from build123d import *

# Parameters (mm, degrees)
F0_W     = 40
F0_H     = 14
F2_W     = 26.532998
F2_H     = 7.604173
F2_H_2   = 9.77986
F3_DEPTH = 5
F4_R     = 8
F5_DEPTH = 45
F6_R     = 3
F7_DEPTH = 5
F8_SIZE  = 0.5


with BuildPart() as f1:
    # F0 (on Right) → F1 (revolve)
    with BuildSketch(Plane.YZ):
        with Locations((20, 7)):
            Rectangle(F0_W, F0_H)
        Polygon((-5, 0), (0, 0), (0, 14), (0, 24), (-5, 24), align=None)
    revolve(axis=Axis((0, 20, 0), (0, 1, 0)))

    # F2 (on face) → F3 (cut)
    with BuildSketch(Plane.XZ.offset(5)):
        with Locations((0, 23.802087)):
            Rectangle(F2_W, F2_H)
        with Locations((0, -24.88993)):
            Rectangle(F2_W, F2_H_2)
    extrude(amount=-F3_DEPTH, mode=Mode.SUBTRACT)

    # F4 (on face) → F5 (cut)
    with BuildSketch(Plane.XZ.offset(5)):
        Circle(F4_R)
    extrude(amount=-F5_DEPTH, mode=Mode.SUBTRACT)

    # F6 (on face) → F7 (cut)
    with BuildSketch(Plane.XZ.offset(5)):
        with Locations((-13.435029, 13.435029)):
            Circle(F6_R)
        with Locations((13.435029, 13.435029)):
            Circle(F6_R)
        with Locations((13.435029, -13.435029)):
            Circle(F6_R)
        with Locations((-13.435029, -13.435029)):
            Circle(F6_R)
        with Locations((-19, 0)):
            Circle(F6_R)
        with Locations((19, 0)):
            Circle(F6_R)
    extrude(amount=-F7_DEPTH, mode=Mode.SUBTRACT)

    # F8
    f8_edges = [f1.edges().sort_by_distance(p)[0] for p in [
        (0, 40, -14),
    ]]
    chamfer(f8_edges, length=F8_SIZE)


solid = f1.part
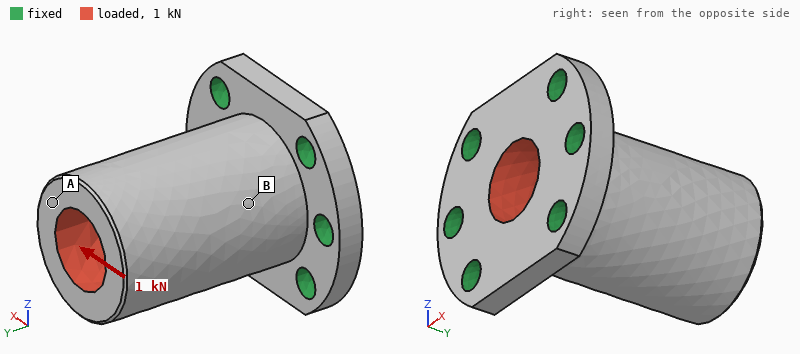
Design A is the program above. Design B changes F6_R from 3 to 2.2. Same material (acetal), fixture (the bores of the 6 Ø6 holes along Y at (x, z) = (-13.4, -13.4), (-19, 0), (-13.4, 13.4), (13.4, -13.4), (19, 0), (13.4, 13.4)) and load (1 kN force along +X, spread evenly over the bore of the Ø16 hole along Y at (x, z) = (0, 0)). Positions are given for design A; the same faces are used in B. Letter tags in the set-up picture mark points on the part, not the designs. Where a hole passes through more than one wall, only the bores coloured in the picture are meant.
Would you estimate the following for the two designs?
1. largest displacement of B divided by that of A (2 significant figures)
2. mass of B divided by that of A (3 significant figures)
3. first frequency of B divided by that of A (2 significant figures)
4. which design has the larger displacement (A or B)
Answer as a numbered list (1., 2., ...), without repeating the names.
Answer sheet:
1. 1.1
2. 1.02
3. 0.93
4. B
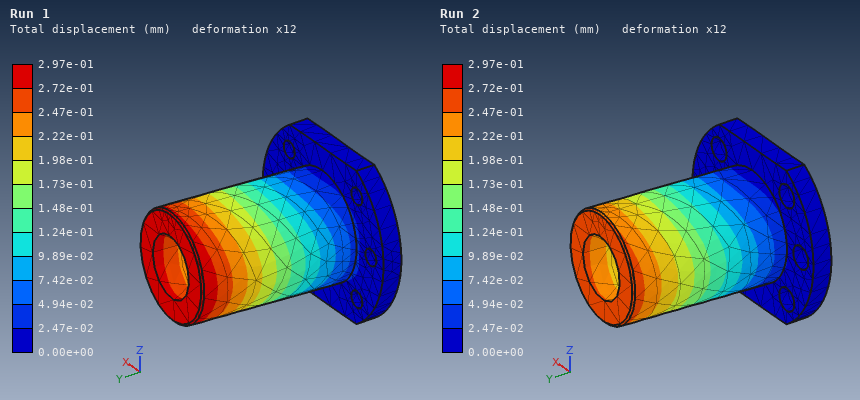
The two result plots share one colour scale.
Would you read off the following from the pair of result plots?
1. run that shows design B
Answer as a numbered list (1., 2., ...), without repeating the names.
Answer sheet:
1. Run 1
